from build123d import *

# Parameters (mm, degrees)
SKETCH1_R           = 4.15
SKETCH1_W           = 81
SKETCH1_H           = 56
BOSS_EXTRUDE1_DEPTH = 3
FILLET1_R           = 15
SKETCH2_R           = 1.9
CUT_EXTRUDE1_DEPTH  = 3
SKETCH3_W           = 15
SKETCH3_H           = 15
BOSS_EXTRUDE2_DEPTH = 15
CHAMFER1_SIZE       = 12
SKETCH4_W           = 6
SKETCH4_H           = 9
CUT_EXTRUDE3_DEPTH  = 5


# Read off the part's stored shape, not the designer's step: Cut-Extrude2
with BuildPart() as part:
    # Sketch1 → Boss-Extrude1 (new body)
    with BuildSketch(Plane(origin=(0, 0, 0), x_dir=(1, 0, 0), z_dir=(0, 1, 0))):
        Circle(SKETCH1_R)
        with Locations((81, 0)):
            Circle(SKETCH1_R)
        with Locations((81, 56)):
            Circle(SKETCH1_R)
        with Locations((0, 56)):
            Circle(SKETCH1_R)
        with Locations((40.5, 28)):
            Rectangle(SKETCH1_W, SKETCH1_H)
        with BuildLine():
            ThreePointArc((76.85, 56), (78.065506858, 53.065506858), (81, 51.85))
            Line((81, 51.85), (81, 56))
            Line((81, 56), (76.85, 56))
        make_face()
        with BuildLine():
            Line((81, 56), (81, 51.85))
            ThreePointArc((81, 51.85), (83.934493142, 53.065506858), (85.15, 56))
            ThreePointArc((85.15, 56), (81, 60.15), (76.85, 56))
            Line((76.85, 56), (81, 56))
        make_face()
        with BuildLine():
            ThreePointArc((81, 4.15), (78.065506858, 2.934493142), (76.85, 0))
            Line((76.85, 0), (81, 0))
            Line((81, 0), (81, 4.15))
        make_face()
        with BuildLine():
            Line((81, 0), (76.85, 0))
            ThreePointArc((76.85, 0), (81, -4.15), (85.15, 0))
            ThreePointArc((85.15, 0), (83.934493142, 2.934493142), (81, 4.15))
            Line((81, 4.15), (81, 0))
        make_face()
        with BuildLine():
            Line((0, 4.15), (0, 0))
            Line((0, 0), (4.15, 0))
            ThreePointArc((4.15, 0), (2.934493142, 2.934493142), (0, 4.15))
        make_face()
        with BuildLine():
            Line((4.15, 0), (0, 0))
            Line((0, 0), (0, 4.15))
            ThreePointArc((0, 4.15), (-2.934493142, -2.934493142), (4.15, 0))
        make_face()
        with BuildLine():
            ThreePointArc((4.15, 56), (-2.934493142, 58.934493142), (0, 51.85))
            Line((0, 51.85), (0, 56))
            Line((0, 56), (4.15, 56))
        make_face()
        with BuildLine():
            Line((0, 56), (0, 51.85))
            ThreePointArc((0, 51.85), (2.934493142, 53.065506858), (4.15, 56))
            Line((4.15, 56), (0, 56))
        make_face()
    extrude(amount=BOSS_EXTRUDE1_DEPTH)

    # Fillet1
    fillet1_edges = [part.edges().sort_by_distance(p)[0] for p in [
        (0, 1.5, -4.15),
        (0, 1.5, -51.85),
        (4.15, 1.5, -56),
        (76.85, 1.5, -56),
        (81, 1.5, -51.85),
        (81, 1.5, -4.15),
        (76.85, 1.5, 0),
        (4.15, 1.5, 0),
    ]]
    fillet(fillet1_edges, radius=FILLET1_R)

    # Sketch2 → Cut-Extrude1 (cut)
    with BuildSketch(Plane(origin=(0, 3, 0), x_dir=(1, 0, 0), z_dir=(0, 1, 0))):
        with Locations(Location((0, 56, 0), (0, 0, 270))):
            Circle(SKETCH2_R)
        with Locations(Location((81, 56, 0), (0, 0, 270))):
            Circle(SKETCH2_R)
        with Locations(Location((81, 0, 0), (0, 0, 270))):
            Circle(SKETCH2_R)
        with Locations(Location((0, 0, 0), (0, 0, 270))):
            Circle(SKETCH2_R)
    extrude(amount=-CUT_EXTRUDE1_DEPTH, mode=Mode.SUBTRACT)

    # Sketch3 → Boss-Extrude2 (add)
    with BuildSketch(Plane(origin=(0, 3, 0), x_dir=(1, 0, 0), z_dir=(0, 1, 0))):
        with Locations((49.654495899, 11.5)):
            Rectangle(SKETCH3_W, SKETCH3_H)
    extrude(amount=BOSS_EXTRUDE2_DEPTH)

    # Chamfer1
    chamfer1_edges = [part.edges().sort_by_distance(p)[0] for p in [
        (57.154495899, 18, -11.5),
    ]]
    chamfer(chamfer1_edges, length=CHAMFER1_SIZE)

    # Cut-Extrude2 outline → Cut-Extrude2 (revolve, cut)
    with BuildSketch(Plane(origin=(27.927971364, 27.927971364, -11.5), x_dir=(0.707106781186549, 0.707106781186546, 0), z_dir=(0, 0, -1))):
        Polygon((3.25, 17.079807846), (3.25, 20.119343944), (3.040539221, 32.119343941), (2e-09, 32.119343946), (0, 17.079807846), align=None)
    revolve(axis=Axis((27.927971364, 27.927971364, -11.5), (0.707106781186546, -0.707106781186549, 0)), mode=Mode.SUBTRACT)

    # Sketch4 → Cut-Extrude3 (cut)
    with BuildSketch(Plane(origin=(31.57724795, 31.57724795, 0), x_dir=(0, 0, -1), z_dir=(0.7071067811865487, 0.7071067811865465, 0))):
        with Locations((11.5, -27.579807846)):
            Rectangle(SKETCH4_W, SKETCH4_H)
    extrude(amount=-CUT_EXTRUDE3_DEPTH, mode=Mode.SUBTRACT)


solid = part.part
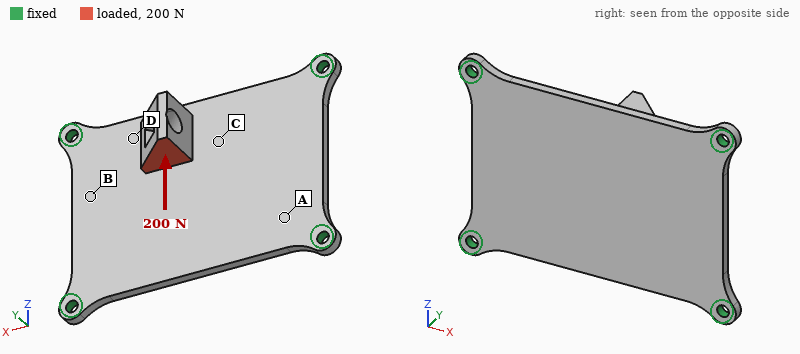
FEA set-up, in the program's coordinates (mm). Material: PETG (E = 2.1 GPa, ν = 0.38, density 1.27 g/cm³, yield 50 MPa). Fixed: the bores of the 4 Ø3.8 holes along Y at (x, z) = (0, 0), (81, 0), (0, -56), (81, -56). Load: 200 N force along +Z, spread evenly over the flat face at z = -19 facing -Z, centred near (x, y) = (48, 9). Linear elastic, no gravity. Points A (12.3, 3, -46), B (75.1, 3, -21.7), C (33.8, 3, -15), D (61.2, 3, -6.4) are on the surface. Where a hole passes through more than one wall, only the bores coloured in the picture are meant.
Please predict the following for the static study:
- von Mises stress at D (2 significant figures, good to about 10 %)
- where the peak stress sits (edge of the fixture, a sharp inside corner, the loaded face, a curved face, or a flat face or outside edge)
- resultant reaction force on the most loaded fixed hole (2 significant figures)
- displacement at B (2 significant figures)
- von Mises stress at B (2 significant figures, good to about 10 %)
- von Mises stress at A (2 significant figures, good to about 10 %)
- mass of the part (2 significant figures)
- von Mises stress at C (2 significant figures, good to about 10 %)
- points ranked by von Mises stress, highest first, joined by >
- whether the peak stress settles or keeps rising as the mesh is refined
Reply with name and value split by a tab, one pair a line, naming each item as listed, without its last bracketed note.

von Mises stress at D	10 MPa
where the peak stress sits	edge of the fixture
resultant reaction force on the most loaded fixed hole	81 N
displacement at B	0.20 mm
von Mises stress at B	5.2 MPa
von Mises stress at A	2.5 MPa
mass of the part	20 g
von Mises stress at C	7.8 MPa
points ranked by von Mises stress, highest first, joined by >	D > C > B > A
whether the peak stress settles or keeps rising as the mesh is refined	keeps rising
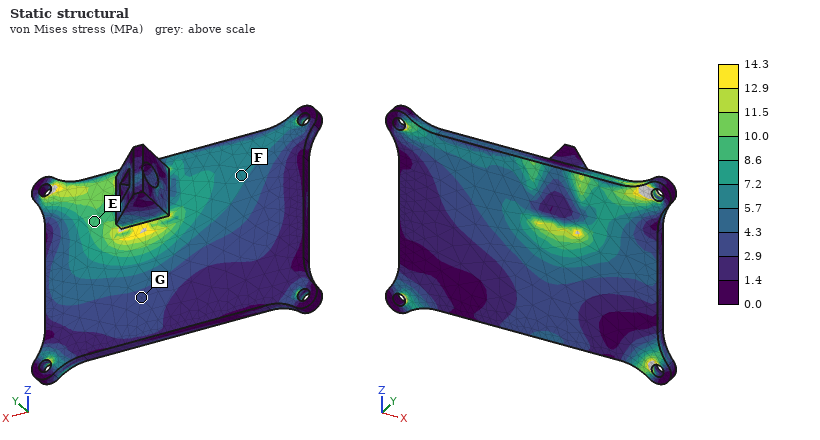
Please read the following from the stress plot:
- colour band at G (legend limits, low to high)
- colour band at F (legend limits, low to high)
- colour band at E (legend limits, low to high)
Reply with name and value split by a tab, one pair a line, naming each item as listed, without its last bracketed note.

colour band at G	2.9 to 4.3 MPa
colour band at F	5.7 to 7.2 MPa
colour band at E	8.6 to 10.0 MPa
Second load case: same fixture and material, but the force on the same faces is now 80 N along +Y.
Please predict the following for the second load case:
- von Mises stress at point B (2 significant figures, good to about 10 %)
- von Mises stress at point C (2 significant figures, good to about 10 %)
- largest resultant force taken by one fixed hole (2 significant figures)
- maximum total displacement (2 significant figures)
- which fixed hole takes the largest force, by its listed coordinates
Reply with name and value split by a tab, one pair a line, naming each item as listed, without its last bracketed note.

von Mises stress at point B	3.8 MPa
von Mises stress at point C	8.3 MPa
largest resultant force taken by one fixed hole	35 N
maximum total displacement	1.2 mm
which fixed hole takes the largest force, by its listed coordinates	(81, 0)
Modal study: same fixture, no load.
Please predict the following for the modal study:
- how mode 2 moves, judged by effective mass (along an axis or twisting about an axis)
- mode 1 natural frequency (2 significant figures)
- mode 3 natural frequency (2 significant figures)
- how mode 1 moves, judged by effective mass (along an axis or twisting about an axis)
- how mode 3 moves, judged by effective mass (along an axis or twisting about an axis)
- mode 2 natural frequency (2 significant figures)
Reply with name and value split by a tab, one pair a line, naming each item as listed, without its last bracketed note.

how mode 2 moves, judged by effective mass	twisting about X
mode 1 natural frequency	430 Hz
mode 3 natural frequency	1100 Hz
how mode 1 moves, judged by effective mass	along Y
how mode 3 moves, judged by effective mass	twisting about Z
mode 2 natural frequency	740 Hz
